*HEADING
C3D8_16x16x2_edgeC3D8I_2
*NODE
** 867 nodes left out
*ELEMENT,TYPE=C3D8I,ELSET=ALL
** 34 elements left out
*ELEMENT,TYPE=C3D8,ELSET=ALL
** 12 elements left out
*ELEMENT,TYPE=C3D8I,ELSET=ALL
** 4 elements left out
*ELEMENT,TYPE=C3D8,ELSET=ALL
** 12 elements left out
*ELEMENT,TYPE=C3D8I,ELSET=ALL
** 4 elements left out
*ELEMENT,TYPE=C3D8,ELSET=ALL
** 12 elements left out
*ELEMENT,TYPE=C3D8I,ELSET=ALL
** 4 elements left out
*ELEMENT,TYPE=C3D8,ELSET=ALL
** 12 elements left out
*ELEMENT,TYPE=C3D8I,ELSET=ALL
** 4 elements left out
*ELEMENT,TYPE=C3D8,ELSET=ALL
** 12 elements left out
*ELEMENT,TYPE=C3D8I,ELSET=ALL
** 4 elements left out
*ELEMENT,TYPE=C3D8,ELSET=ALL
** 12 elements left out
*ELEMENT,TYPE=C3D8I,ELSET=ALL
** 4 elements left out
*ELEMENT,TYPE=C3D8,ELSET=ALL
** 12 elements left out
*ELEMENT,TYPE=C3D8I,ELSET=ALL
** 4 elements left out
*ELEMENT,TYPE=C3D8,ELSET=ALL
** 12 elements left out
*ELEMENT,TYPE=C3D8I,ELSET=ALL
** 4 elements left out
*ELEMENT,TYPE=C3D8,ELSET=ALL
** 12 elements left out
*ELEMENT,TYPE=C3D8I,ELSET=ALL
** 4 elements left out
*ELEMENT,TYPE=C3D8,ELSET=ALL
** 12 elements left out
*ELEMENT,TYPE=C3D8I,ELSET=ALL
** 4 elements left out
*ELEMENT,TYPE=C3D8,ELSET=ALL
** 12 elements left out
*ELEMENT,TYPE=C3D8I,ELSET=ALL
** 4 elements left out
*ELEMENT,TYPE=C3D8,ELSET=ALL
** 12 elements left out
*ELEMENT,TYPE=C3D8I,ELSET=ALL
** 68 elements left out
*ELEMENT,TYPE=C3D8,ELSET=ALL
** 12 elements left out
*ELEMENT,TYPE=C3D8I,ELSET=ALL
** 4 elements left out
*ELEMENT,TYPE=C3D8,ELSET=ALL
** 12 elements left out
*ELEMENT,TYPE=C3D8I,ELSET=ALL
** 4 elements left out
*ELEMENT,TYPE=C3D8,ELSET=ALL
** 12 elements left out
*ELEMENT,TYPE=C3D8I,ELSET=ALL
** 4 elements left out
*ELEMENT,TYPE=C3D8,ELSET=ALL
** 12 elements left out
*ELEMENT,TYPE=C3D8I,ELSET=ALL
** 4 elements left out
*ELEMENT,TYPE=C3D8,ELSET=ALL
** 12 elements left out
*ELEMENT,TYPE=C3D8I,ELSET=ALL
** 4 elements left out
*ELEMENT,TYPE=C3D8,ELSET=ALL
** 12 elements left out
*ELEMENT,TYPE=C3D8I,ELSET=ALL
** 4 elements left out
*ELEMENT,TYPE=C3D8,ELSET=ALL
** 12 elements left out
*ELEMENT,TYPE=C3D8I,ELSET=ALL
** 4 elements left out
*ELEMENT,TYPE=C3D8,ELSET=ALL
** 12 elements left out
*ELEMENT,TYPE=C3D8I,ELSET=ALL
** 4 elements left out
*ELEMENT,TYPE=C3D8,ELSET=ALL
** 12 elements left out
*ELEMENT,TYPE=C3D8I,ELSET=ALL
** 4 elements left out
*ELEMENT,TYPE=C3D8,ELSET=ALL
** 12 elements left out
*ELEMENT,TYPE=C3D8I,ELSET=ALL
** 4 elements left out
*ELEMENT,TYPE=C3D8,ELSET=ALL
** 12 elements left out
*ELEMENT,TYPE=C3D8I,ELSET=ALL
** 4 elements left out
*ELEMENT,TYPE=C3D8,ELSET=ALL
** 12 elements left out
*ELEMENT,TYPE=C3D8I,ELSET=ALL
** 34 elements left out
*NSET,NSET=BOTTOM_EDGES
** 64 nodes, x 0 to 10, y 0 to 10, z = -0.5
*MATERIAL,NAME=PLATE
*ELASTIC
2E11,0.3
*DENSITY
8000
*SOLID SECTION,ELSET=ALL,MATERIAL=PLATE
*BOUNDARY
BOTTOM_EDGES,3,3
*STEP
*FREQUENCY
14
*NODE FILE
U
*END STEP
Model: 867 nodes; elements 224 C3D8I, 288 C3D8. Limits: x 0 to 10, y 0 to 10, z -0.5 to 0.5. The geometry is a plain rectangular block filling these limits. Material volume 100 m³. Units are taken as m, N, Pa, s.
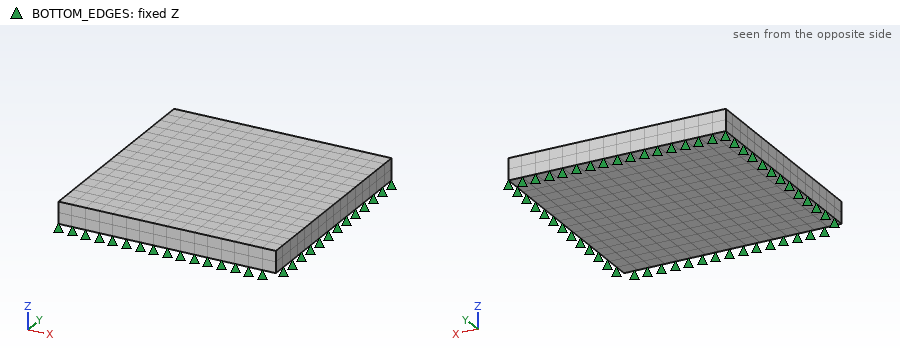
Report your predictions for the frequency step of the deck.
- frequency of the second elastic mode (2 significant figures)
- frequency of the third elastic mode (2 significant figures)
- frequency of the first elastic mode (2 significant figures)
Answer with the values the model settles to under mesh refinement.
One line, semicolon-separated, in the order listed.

100 Hz; 100 Hz; 43 Hz
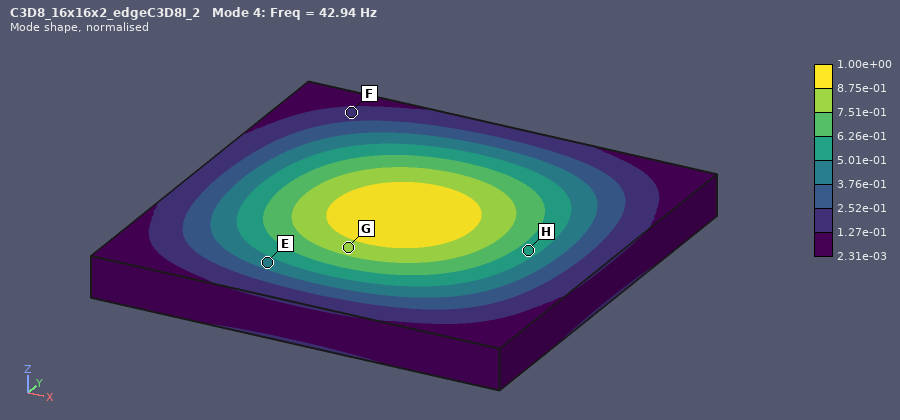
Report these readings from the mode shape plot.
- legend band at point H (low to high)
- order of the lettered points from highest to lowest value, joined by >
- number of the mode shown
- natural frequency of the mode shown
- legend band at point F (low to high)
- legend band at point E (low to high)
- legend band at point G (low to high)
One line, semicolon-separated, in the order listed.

5.01e-01 to 6.26e-01; G > H > E > F; 4; 42.94 Hz; 1.27e-01 to 2.52e-01; 3.76e-01 to 5.01e-01; 7.51e-01 to 8.75e-01
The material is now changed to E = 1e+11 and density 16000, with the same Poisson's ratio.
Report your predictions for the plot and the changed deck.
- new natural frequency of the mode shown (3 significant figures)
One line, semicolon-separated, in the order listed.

21.5 Hz
